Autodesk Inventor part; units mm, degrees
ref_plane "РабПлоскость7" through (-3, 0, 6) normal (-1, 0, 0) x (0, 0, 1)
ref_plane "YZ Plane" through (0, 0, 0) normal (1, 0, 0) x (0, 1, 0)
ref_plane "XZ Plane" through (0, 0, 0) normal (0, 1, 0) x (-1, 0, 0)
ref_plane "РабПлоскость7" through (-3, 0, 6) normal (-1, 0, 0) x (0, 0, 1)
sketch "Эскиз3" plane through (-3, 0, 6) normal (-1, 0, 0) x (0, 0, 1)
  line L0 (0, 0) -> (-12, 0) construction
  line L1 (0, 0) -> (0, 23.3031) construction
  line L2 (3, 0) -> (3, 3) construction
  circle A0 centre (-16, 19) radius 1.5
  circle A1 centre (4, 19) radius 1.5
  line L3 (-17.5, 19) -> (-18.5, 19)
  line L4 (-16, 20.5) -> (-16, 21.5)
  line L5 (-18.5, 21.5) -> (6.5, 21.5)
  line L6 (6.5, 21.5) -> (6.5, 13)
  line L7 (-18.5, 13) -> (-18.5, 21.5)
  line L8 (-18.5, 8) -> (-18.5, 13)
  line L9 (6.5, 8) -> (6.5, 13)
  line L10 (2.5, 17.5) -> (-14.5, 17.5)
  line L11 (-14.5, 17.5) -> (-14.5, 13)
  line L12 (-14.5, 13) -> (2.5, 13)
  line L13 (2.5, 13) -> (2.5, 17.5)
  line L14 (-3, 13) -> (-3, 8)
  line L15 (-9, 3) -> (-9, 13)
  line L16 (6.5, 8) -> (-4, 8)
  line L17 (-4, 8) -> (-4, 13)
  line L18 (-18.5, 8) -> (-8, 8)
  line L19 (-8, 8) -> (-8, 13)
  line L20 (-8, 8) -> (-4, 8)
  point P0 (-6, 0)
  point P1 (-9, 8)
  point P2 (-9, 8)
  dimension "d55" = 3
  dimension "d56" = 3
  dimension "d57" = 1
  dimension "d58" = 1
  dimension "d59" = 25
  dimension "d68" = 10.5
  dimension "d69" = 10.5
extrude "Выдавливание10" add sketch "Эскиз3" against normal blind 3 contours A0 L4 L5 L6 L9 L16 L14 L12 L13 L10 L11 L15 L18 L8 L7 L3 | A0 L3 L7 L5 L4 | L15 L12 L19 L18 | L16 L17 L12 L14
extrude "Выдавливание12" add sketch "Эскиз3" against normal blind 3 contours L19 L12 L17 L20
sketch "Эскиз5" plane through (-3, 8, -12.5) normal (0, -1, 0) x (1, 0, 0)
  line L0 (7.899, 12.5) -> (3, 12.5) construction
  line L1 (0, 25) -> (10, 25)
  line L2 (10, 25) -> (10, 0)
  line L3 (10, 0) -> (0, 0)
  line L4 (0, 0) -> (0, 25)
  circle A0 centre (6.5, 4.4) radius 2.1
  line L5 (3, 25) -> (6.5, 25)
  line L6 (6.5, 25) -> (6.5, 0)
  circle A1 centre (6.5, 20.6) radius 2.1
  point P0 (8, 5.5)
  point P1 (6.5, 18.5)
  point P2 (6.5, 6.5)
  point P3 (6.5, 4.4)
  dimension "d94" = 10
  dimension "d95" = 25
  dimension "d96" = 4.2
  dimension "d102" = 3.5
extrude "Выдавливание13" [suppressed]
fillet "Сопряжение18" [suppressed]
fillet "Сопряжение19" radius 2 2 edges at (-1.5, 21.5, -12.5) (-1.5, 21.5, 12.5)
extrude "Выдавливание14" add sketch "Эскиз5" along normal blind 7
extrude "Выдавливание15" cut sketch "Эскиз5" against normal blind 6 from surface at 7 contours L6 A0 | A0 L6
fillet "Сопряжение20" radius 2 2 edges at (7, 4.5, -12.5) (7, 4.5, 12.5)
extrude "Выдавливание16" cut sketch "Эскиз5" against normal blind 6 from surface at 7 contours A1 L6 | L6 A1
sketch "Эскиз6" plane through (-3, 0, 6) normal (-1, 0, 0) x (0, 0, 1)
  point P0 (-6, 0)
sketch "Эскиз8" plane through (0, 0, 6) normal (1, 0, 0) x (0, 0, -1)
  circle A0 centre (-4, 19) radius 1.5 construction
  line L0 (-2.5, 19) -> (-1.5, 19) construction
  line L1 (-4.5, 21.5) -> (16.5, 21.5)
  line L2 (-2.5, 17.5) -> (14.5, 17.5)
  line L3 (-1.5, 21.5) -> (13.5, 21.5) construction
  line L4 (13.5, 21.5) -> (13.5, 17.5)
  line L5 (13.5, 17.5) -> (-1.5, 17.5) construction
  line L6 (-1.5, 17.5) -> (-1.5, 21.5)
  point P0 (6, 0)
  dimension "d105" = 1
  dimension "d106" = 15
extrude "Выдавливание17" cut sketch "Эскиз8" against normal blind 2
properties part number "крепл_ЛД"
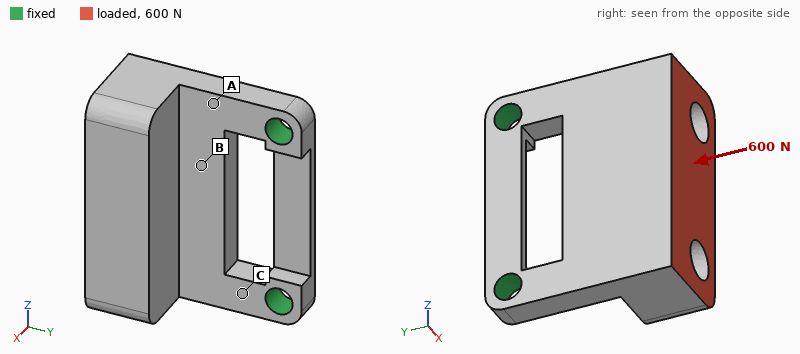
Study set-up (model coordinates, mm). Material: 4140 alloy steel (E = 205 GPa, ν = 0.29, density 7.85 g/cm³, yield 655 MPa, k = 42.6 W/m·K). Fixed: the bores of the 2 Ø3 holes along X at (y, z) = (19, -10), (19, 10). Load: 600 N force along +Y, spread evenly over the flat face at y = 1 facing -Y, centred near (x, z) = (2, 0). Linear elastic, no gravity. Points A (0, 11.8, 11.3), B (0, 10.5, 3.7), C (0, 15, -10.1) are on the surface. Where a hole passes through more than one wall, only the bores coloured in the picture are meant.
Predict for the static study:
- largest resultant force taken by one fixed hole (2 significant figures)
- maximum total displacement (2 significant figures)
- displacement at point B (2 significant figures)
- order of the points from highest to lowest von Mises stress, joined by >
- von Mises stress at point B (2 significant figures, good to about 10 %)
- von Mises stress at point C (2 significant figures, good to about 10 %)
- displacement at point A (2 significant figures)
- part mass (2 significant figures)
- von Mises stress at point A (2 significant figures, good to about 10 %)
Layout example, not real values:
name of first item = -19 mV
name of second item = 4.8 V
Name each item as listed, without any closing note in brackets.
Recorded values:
largest resultant force taken by one fixed hole = 300 N
maximum total displacement = 71 µm
displacement at point B = 16 µm
order of the points from highest to lowest von Mises stress, joined by > = C > A > B
von Mises stress at point B = 29 MPa
von Mises stress at point C = 190 MPa
displacement at point A = 11 µm
part mass = 17 g
von Mises stress at point A = 150 MPa
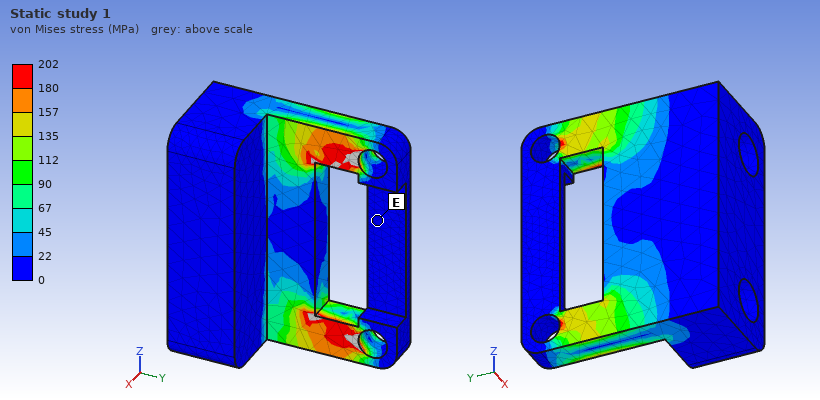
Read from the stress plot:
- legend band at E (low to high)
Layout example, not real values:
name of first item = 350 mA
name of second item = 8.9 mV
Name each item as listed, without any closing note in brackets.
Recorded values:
legend band at E = 0 to 22 MPa
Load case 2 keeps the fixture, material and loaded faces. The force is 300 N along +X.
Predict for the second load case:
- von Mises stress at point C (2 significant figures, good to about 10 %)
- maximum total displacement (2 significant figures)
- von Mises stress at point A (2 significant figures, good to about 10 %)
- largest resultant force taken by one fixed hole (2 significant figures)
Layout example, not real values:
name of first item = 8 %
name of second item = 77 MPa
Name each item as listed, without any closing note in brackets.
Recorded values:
von Mises stress at point C = 360 MPa
maximum total displacement = 0.14 mm
von Mises stress at point A = 220 MPa
largest resultant force taken by one fixed hole = 150 N
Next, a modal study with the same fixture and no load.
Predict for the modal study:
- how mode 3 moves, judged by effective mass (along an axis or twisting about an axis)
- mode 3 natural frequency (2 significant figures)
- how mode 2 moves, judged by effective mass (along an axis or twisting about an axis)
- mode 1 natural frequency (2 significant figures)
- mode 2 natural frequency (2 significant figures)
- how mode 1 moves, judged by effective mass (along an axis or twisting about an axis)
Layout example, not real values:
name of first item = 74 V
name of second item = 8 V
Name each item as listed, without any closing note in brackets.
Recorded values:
how mode 3 moves, judged by effective mass = along Z
mode 3 natural frequency = 14 kHz
how mode 2 moves, judged by effective mass = along Z
mode 1 natural frequency = 2800 Hz
mode 2 natural frequency = 9200 Hz
how mode 1 moves, judged by effective mass = along X
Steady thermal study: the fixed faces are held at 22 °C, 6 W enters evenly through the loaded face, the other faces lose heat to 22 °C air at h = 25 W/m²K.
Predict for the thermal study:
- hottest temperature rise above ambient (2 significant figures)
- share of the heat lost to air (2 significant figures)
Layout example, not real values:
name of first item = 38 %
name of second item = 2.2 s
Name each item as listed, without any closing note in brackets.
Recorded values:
hottest temperature rise above ambient = 47 K
share of the heat lost to air = 21 %
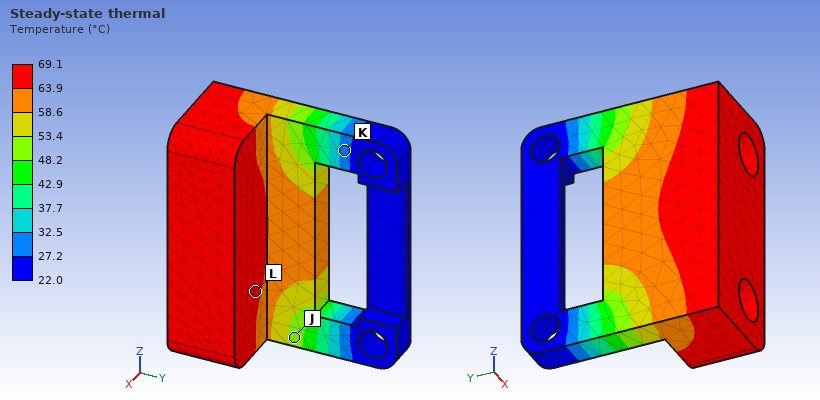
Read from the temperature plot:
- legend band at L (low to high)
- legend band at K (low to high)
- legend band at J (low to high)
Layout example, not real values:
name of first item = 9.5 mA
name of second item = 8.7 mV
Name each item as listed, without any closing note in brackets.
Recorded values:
legend band at L = 63.9 to 69.1 °C
legend band at K = 27.2 to 32.5 °C
legend band at J = 48.2 to 53.4 °C
